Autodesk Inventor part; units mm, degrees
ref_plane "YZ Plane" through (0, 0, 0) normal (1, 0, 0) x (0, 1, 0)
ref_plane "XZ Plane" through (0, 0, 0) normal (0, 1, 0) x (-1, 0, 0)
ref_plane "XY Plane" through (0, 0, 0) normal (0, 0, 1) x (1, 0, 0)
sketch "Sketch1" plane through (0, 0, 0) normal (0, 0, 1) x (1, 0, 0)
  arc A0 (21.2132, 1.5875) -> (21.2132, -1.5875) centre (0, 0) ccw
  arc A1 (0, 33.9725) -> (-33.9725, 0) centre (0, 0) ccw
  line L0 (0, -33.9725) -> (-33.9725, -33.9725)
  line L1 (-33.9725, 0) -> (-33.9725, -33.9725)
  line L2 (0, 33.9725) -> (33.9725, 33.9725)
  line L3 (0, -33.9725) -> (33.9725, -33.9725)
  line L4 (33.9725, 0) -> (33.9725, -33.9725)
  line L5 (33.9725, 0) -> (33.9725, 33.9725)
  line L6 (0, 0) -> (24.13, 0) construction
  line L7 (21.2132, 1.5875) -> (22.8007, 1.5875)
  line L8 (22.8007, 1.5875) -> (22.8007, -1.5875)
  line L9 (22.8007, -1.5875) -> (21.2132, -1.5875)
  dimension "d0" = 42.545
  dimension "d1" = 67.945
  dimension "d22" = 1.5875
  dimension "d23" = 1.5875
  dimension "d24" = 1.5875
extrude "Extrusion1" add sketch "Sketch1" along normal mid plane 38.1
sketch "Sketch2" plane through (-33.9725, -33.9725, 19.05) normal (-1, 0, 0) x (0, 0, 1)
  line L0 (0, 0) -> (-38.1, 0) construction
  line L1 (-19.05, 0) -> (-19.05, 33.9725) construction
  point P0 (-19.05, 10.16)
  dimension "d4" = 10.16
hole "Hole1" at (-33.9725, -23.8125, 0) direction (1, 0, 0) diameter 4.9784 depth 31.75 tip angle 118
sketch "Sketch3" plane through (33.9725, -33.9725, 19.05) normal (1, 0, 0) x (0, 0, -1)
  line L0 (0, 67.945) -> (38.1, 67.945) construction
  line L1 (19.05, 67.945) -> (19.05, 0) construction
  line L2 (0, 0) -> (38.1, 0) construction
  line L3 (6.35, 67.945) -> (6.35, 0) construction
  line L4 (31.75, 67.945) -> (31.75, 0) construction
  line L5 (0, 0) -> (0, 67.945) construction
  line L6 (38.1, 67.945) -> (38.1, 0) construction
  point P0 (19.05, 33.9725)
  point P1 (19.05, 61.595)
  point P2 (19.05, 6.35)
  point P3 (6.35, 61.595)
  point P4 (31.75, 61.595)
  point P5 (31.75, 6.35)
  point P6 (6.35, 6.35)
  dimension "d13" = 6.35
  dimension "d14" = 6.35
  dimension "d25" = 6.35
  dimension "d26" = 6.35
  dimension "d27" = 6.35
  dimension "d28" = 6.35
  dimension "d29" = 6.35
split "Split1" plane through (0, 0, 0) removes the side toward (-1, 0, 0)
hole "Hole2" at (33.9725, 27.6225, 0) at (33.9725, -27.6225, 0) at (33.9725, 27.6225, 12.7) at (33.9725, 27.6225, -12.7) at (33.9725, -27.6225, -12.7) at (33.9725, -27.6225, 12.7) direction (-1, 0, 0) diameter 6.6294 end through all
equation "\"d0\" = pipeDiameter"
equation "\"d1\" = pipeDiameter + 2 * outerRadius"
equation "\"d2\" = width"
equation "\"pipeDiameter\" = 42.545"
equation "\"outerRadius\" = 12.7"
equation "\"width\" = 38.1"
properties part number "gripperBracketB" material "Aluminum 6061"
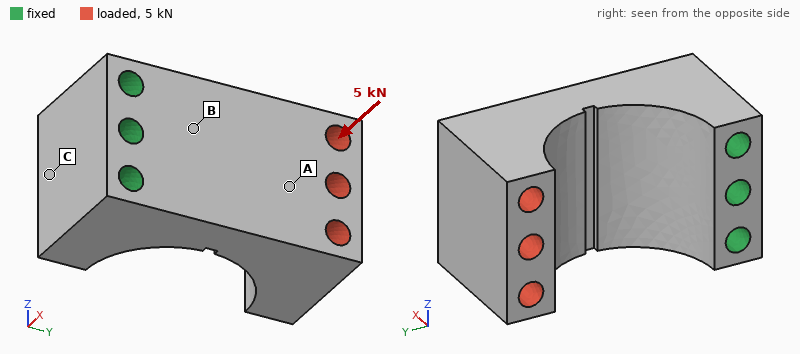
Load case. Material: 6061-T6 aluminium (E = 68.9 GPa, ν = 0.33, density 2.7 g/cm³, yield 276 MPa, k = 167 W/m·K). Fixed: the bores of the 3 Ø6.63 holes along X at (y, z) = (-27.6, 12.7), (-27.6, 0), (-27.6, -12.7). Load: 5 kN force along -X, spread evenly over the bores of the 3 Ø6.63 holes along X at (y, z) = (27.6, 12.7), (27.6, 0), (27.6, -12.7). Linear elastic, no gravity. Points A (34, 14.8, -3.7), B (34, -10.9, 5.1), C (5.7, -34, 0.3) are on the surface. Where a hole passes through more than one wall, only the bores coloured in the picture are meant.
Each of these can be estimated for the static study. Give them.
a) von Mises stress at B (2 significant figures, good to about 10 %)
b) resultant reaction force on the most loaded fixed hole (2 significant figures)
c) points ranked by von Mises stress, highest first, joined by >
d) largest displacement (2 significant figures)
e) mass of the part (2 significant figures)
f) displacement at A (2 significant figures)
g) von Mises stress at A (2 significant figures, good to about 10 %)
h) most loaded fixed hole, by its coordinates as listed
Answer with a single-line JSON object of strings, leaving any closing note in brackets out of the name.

{"von Mises stress at B": "130 MPa", "resultant reaction force on the most loaded fixed hole": "2.6 kN", "points ranked by von Mises stress, highest first, joined by >": "B > A > C", "largest displacement": "0.46 mm", "mass of the part": "140 g", "displacement at A": "0.20 mm", "von Mises stress at A": "41 MPa", "most loaded fixed hole, by its coordinates as listed": "(-27.6, 0)"}
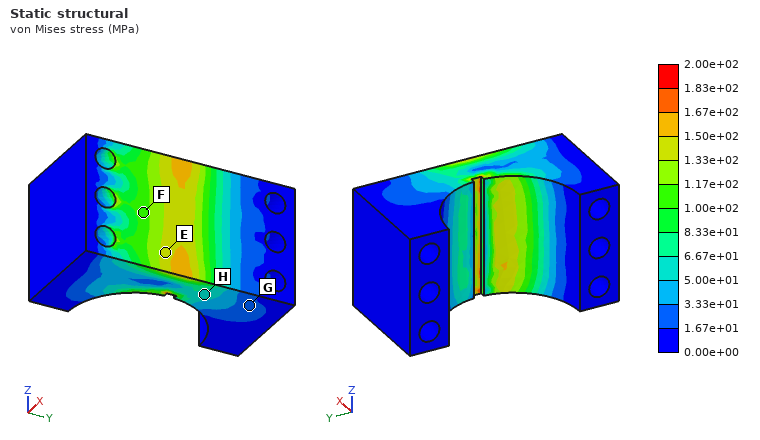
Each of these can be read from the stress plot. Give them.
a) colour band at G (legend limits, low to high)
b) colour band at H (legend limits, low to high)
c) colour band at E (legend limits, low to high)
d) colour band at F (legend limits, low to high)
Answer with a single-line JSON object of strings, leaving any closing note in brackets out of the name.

{"colour band at G": "1.67e+01 to 3.33e+01 MPa", "colour band at H": "5.00e+01 to 6.67e+01 MPa", "colour band at E": "1.33e+02 to 1.50e+02 MPa", "colour band at F": "1.00e+02 to 1.17e+02 MPa"}
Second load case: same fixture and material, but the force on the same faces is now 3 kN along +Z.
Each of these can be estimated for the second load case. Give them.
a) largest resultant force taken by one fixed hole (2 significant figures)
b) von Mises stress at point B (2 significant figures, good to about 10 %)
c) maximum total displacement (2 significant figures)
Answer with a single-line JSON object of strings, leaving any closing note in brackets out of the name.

{"largest resultant force taken by one fixed hole": "5.7 kN", "von Mises stress at point B": "15 MPa", "maximum total displacement": "92 µm"}
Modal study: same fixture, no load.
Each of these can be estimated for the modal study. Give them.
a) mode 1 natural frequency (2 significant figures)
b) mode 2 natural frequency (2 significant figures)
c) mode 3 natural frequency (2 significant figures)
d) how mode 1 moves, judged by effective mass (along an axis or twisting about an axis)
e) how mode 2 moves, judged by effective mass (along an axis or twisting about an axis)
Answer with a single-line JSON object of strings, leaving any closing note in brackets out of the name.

{"mode 1 natural frequency": "2700 Hz", "mode 2 natural frequency": "4800 Hz", "mode 3 natural frequency": "7900 Hz", "how mode 1 moves, judged by effective mass": "along X", "how mode 2 moves, judged by effective mass": "along Z"}
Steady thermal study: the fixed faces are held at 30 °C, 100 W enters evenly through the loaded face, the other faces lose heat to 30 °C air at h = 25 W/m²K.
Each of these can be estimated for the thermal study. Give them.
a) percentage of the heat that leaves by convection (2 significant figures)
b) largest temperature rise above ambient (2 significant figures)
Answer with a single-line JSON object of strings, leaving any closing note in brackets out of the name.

{"percentage of the heat that leaves by convection": "7.3 %", "largest temperature rise above ambient": "55 K"}
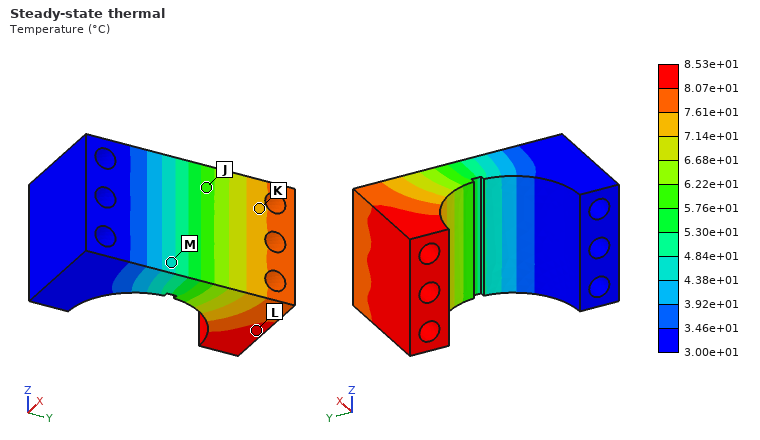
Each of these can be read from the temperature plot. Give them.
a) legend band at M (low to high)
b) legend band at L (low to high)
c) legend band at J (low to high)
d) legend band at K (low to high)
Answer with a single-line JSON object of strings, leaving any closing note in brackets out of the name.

{"legend band at M": "4.38e+01 to 4.84e+01 °C", "legend band at L": "8.07e+01 to 8.53e+01 °C", "legend band at J": "5.76e+01 to 6.22e+01 °C", "legend band at K": "7.14e+01 to 7.61e+01 °C"}
